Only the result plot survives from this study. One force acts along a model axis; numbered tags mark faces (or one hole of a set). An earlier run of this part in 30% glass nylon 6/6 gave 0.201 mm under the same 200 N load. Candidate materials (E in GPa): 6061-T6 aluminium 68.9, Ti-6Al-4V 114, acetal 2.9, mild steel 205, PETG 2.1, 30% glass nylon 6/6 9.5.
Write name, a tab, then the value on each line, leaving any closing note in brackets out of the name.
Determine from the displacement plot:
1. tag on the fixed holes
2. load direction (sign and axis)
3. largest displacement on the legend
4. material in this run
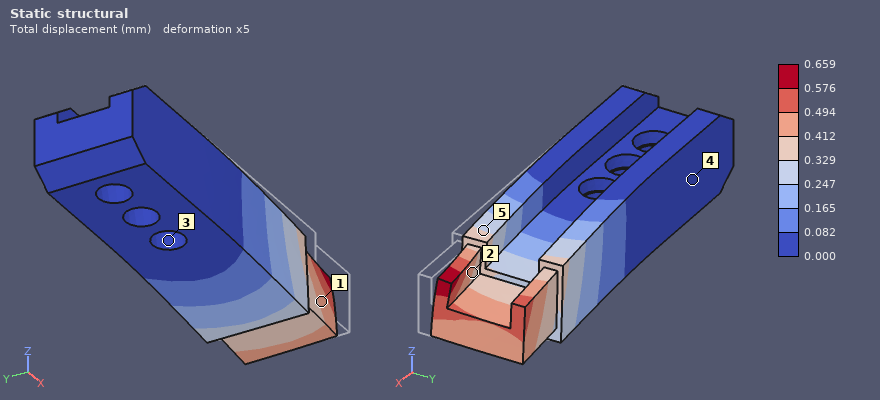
tag on the fixed holes	3
load direction	+Y
largest displacement on the legend	0.659 mm
material in this run	acetal
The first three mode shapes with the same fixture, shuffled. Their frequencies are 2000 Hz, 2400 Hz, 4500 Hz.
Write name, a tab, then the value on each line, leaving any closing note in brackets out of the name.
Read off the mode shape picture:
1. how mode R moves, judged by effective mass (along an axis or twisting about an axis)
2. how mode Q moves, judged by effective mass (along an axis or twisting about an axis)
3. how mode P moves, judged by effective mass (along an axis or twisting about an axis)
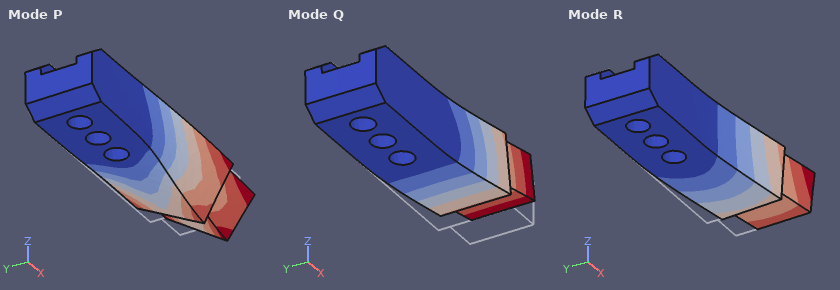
how mode R moves, judged by effective mass	along Y
how mode Q moves, judged by effective mass	along Z
how mode P moves, judged by effective mass	twisting about X
